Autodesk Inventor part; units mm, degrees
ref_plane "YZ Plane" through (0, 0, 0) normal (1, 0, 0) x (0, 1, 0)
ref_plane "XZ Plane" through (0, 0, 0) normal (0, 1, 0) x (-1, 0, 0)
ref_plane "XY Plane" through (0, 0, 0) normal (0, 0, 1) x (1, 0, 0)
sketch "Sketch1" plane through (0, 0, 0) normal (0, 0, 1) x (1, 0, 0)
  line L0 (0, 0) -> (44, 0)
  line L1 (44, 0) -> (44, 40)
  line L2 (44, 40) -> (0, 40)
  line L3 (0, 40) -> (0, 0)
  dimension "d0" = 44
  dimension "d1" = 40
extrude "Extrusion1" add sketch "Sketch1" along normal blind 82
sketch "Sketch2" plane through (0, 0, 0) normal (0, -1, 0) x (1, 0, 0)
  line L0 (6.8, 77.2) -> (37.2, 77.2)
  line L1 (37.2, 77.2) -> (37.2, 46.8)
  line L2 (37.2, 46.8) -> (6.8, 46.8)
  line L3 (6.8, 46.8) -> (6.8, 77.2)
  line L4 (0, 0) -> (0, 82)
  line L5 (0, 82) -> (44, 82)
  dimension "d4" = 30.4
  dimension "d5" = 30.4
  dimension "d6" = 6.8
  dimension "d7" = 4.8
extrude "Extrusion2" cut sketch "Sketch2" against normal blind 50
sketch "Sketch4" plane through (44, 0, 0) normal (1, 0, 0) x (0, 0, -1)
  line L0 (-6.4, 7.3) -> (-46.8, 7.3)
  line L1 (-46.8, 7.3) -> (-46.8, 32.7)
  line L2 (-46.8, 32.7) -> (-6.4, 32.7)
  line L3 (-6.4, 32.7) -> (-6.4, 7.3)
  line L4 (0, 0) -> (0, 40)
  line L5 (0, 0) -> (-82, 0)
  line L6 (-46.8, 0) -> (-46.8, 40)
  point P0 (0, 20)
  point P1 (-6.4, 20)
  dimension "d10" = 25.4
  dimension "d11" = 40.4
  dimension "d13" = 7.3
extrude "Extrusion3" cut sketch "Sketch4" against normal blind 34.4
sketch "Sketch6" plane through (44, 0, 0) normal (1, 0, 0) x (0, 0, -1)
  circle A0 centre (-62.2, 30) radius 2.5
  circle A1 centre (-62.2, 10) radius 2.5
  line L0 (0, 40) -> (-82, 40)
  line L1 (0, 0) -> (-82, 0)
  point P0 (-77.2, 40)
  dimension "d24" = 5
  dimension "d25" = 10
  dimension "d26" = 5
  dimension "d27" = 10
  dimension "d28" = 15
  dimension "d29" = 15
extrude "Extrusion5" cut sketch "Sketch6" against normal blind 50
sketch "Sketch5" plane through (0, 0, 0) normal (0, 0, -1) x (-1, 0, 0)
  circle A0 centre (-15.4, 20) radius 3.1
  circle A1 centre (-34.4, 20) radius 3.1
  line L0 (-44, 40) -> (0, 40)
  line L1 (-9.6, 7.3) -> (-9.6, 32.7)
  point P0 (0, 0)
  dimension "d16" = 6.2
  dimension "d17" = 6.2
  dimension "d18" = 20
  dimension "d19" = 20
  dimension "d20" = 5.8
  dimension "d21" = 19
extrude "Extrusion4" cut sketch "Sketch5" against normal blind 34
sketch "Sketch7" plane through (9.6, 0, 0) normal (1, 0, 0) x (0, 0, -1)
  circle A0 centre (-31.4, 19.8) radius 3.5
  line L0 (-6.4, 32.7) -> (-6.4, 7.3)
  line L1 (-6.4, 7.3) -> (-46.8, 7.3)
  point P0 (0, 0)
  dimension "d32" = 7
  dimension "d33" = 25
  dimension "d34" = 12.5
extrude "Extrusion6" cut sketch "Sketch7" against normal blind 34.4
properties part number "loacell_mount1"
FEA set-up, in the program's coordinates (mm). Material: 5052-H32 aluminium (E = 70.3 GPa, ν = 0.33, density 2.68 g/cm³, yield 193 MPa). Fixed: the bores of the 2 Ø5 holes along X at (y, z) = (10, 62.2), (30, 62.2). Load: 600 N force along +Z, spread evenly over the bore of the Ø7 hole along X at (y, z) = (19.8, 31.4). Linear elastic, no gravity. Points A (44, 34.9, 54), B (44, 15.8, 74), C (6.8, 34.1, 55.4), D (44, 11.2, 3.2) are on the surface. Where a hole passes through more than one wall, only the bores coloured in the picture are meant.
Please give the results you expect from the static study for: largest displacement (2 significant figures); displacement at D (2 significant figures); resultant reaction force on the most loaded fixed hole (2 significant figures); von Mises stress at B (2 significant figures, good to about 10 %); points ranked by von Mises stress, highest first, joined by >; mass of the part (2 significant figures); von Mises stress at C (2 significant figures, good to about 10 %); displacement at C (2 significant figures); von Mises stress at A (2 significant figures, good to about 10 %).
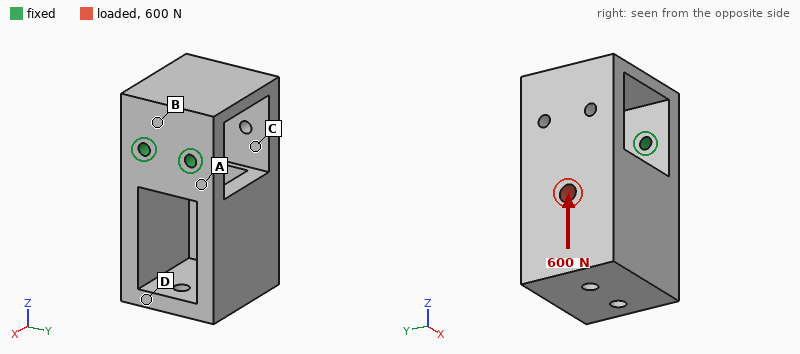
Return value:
0.18 mm
0.14 mm
310 N
19 MPa
A > B > C > D
190 g
12 MPa
0.095 mm
26 MPa
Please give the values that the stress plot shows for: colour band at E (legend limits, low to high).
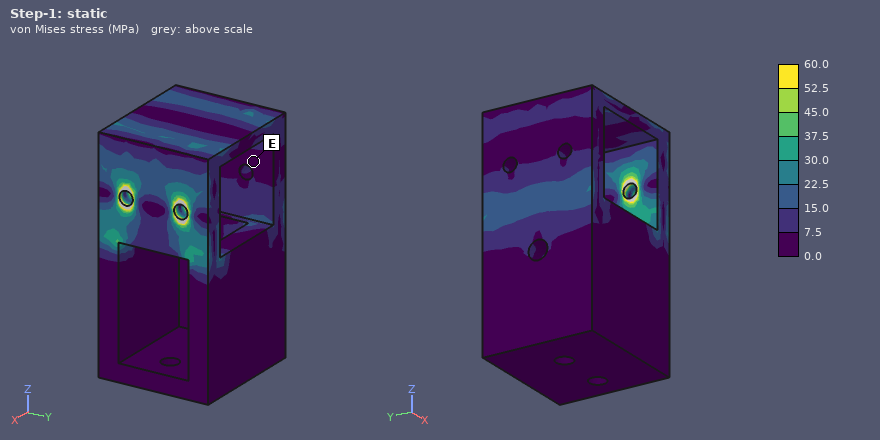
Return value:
0.0 to 7.5 MPa
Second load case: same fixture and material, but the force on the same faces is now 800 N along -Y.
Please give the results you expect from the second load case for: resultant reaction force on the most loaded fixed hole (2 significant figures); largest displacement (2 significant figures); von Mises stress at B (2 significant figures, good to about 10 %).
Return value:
1.5 kN
96 µm
18 MPa
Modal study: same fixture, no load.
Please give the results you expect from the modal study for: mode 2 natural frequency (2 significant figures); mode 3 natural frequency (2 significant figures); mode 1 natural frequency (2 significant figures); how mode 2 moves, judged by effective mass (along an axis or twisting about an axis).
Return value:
1400 Hz
2700 Hz
830 Hz
along Y
